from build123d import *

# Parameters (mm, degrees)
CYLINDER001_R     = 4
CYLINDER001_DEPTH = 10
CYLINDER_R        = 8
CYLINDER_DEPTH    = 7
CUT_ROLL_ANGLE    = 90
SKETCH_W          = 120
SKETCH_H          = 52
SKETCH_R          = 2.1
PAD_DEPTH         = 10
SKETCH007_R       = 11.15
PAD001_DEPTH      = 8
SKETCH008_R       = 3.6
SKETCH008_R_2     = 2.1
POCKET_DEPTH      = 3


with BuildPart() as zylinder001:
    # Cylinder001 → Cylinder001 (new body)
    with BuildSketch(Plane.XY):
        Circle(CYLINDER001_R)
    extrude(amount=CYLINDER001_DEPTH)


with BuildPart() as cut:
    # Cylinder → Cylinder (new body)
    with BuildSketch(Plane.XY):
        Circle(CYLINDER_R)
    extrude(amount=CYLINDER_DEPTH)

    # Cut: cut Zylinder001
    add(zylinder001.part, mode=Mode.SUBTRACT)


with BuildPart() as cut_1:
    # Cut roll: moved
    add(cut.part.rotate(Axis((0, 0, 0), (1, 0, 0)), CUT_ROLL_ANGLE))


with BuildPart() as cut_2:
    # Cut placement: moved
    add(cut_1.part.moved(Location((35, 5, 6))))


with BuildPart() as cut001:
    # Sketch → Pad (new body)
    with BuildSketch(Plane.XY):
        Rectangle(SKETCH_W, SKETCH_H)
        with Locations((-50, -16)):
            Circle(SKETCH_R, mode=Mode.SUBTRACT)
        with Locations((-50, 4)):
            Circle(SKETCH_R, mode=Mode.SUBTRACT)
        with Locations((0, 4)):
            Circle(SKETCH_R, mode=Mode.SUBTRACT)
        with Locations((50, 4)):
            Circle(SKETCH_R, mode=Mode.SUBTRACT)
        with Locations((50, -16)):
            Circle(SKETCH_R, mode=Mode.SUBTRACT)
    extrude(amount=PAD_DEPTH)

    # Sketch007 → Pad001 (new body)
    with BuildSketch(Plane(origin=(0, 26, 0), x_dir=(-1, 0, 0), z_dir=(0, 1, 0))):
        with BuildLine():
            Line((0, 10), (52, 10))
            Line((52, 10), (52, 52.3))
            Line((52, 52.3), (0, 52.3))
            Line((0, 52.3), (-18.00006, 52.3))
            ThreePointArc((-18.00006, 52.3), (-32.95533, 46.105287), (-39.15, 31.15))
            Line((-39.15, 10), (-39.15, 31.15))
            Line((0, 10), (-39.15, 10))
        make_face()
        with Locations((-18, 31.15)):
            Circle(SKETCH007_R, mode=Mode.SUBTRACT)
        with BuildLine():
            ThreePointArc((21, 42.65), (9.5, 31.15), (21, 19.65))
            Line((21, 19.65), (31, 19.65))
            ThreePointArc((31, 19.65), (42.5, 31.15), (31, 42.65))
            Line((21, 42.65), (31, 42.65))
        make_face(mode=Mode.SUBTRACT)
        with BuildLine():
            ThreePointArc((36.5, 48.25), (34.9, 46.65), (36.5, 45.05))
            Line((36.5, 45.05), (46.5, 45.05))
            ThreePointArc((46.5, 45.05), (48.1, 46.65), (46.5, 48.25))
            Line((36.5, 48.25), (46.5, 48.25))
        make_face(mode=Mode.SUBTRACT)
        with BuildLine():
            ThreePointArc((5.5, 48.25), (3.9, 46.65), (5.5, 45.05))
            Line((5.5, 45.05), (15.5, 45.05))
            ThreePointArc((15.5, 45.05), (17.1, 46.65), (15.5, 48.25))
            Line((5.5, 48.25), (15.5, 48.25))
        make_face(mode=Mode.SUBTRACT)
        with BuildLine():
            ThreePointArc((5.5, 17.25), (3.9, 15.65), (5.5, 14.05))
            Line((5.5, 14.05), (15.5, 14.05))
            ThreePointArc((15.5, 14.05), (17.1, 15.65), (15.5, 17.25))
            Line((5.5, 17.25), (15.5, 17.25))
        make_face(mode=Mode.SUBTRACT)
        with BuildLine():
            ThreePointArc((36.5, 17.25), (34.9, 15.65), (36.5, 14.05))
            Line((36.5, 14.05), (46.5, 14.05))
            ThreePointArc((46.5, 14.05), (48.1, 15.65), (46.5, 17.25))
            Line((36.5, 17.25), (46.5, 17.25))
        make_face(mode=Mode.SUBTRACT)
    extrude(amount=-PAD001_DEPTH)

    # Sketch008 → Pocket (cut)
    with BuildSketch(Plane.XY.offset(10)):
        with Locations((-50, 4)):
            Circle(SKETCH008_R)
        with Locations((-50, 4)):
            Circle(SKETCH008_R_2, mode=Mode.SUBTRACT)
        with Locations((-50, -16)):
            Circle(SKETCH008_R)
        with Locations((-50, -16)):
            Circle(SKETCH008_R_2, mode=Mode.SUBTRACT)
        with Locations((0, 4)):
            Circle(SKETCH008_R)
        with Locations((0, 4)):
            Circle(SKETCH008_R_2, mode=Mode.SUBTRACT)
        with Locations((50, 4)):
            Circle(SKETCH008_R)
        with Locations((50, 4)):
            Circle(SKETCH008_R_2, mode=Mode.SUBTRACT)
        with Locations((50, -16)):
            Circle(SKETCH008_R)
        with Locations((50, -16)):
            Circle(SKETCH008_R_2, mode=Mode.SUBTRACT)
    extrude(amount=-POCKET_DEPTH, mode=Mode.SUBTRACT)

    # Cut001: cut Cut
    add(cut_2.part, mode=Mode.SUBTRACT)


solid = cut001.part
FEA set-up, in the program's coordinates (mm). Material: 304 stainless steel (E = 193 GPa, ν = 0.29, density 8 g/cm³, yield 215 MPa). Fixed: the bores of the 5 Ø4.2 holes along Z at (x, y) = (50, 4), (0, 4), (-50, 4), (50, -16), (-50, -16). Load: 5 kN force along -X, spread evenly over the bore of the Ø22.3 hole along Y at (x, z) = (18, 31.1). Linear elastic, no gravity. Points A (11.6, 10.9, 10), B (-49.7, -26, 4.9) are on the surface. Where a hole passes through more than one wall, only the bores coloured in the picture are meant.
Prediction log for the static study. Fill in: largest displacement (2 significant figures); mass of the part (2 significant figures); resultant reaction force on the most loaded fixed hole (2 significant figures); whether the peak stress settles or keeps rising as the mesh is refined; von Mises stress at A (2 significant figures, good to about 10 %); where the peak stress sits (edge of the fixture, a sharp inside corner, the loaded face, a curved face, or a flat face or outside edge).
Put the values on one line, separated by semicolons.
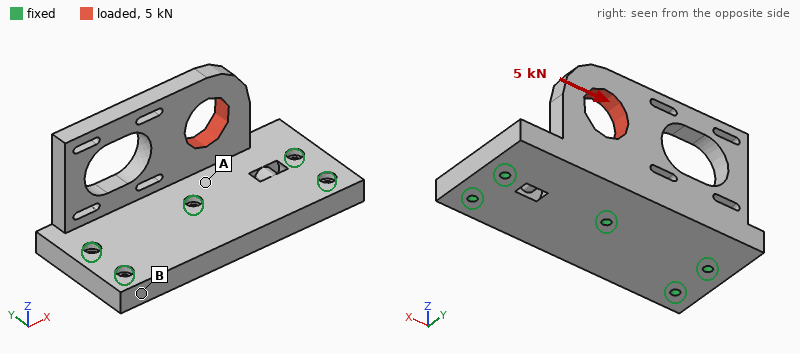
28 µm; 650 g; 2.4 kN; keeps rising; 21 MPa; edge of the fixture
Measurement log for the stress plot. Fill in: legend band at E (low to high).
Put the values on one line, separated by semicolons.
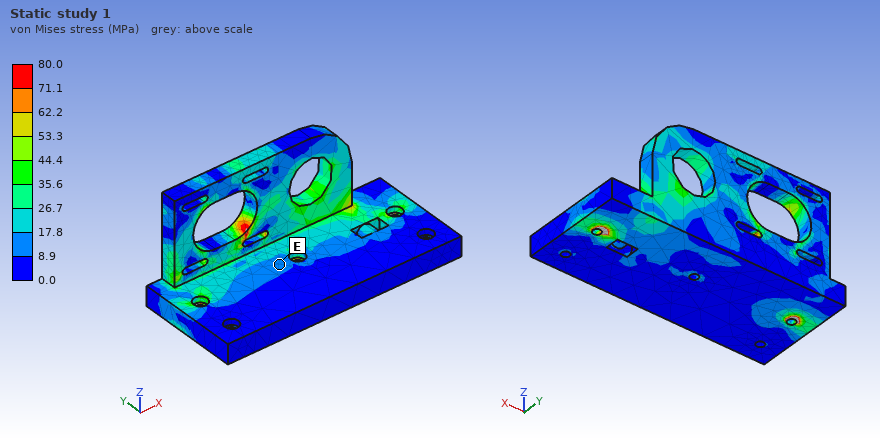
8.9 to 17.8 MPa
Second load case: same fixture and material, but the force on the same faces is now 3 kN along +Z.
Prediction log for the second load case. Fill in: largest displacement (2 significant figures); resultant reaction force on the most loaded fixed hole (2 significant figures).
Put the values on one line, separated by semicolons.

39 µm; 2.0 kN
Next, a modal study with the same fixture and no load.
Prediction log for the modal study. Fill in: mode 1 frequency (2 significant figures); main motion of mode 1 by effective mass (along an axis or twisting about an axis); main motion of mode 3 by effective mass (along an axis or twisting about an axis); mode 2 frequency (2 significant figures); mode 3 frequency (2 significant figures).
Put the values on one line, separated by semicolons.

2000 Hz; along Y; along Z; 3500 Hz; 5700 Hz
